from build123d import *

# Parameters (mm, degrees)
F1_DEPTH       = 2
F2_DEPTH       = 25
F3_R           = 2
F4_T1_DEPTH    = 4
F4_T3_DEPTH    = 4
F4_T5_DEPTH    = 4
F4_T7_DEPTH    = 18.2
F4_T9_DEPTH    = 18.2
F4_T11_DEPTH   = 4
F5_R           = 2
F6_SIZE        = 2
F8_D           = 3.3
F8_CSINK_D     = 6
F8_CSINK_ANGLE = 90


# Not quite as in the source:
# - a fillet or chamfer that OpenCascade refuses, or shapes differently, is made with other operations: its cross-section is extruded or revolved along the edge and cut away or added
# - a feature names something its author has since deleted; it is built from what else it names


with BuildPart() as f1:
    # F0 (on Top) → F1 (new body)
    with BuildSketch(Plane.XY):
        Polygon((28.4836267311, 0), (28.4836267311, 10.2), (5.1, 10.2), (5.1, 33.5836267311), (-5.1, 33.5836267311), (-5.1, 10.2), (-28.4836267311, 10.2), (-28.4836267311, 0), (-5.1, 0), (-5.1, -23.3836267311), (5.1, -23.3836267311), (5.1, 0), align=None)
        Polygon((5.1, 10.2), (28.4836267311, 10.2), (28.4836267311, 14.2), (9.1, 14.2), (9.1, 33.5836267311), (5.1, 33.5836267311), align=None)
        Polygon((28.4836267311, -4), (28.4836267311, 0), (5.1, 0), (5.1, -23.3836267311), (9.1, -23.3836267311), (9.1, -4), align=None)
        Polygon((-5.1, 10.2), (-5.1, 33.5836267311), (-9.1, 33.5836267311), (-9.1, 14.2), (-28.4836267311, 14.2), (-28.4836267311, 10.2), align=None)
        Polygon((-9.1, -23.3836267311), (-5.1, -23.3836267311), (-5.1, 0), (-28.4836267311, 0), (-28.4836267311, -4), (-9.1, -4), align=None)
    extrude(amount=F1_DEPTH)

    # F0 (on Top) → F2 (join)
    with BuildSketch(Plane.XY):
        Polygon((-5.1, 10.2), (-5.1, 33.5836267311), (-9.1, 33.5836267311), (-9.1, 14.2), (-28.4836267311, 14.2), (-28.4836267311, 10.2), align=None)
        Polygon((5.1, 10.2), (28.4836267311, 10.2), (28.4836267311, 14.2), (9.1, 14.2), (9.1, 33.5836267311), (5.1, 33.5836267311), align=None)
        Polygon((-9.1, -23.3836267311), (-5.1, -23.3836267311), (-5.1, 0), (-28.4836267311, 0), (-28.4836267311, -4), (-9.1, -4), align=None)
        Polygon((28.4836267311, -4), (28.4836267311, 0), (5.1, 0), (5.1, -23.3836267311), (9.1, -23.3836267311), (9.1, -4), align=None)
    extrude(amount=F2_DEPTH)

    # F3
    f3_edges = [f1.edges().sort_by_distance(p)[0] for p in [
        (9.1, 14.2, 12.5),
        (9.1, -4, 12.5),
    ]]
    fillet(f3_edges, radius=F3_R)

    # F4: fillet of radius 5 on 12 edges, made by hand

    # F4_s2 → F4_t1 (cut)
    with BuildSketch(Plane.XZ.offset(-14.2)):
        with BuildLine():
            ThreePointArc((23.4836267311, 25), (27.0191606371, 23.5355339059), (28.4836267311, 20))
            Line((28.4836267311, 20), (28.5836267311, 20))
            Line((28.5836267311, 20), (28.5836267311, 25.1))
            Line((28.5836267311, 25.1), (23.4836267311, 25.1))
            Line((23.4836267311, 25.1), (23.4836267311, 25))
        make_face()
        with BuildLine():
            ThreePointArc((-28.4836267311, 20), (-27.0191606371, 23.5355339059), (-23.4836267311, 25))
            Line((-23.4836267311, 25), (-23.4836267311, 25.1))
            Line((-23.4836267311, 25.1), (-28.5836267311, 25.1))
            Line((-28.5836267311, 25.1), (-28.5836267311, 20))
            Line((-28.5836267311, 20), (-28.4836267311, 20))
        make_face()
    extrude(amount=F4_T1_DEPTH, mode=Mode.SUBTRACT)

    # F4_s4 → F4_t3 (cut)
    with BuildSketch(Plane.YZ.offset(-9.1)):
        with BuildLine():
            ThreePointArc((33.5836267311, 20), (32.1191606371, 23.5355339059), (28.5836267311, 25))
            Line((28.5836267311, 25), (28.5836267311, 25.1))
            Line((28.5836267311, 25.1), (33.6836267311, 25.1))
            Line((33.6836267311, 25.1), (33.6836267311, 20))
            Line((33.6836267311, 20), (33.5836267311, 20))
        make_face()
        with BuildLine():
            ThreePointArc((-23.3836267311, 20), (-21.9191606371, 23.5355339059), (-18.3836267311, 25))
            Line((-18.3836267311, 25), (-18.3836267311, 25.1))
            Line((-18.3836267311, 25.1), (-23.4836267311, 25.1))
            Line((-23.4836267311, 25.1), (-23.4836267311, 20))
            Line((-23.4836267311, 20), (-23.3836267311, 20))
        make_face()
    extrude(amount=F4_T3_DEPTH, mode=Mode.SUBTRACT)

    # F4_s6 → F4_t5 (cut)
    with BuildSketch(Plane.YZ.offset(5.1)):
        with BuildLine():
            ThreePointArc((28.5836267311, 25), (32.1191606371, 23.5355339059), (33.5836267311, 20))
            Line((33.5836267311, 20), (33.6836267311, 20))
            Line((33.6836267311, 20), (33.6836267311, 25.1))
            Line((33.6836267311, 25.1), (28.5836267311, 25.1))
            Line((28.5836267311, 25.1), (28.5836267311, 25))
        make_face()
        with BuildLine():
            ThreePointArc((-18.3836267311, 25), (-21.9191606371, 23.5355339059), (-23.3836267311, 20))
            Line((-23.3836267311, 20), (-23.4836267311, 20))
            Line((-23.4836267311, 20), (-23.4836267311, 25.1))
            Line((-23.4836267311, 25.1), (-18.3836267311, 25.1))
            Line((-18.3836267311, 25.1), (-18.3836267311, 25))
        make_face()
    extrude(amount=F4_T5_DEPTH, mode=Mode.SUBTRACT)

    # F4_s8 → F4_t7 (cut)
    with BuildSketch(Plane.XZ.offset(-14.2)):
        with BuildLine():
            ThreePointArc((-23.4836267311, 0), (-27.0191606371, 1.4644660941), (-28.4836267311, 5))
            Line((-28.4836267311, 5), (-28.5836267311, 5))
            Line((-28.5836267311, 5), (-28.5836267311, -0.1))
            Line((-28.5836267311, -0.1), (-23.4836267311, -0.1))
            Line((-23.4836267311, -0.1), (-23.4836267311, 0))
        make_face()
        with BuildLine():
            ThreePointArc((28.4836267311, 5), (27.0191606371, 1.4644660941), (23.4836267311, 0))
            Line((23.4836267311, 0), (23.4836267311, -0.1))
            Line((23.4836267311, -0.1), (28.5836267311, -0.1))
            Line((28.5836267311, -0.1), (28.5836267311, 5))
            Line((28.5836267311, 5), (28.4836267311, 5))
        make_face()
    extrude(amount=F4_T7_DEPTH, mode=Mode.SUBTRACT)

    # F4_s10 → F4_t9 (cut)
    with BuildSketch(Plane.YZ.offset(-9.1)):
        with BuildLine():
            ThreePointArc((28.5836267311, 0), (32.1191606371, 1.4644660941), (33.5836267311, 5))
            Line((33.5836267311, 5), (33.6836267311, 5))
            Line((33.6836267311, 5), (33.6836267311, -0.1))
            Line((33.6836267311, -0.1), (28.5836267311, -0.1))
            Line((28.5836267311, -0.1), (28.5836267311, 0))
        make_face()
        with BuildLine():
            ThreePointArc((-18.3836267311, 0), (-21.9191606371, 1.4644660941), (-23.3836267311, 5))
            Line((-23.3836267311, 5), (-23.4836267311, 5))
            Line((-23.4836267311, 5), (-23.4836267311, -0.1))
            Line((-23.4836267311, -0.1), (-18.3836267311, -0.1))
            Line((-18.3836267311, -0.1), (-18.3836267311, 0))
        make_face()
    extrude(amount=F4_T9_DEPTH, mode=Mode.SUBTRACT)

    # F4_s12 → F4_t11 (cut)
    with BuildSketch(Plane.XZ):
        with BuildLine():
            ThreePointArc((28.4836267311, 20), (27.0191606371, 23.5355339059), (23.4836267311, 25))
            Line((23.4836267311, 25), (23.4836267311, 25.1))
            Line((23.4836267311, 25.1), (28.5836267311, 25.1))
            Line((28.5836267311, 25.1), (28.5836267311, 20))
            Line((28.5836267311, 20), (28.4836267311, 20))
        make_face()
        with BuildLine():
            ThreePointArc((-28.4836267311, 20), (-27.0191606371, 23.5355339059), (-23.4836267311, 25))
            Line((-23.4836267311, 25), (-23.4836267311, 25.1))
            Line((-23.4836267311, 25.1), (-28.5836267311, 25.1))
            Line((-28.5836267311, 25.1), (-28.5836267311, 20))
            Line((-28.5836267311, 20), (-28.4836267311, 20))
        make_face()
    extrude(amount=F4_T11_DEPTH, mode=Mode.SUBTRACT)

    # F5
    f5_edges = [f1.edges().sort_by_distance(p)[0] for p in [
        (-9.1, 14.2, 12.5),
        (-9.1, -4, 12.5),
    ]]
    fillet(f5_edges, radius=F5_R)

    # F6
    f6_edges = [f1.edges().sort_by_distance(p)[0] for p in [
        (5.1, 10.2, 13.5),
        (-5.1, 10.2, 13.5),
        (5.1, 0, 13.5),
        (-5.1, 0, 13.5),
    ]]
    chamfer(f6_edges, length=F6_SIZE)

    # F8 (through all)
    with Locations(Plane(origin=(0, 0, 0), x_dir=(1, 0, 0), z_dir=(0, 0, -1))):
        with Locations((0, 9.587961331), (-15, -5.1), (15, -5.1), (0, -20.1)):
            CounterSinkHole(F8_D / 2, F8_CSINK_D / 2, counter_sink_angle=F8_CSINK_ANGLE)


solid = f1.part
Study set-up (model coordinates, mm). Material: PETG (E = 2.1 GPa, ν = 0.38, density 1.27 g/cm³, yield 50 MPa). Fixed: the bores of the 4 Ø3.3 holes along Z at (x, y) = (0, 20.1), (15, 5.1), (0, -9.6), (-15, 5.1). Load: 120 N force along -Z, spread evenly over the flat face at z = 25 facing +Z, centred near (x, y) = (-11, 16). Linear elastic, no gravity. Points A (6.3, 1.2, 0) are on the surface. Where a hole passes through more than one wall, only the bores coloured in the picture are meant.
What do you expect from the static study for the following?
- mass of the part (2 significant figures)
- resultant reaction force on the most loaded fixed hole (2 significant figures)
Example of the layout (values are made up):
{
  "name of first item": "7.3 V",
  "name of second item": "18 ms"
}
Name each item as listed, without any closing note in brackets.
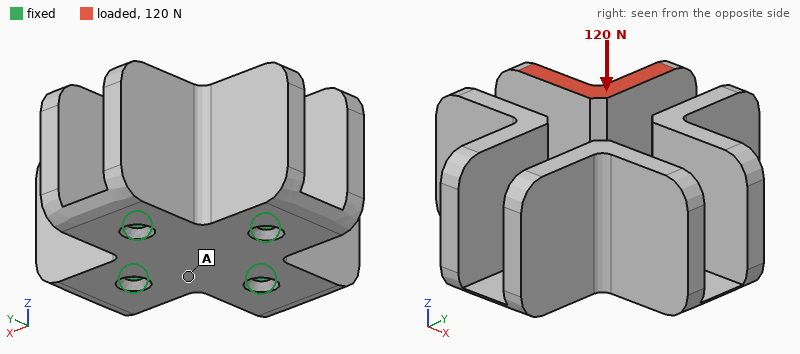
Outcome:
{
  "mass of the part": "23 g",
  "resultant reaction force on the most loaded fixed hole": "72 N"
}
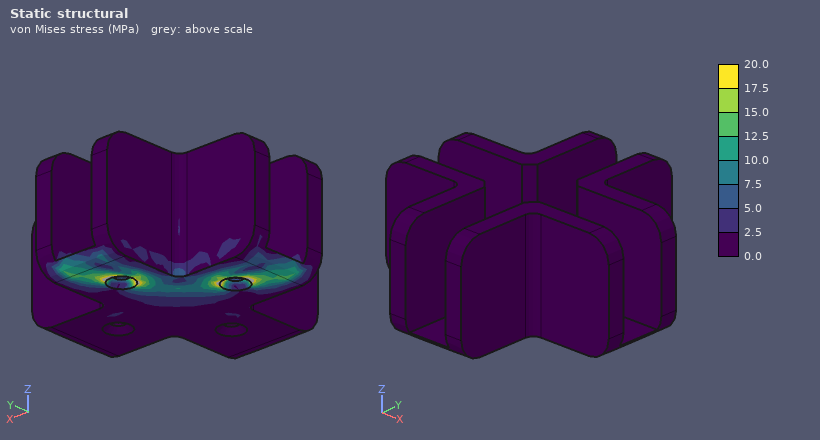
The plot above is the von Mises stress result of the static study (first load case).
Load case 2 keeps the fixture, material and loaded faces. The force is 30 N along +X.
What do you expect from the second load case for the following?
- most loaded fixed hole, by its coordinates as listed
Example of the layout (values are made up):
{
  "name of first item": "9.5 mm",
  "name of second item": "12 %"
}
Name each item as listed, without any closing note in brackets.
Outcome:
{
  "most loaded fixed hole, by its coordinates as listed": "(-15, 5.1)"
}
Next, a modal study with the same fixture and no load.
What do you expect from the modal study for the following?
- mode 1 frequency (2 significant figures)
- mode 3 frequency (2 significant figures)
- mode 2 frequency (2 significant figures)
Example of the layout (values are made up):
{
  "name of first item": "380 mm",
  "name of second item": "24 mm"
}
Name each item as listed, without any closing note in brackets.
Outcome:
{
  "mode 1 frequency": "460 Hz",
  "mode 3 frequency": "590 Hz",
  "mode 2 frequency": "590 Hz"
}
